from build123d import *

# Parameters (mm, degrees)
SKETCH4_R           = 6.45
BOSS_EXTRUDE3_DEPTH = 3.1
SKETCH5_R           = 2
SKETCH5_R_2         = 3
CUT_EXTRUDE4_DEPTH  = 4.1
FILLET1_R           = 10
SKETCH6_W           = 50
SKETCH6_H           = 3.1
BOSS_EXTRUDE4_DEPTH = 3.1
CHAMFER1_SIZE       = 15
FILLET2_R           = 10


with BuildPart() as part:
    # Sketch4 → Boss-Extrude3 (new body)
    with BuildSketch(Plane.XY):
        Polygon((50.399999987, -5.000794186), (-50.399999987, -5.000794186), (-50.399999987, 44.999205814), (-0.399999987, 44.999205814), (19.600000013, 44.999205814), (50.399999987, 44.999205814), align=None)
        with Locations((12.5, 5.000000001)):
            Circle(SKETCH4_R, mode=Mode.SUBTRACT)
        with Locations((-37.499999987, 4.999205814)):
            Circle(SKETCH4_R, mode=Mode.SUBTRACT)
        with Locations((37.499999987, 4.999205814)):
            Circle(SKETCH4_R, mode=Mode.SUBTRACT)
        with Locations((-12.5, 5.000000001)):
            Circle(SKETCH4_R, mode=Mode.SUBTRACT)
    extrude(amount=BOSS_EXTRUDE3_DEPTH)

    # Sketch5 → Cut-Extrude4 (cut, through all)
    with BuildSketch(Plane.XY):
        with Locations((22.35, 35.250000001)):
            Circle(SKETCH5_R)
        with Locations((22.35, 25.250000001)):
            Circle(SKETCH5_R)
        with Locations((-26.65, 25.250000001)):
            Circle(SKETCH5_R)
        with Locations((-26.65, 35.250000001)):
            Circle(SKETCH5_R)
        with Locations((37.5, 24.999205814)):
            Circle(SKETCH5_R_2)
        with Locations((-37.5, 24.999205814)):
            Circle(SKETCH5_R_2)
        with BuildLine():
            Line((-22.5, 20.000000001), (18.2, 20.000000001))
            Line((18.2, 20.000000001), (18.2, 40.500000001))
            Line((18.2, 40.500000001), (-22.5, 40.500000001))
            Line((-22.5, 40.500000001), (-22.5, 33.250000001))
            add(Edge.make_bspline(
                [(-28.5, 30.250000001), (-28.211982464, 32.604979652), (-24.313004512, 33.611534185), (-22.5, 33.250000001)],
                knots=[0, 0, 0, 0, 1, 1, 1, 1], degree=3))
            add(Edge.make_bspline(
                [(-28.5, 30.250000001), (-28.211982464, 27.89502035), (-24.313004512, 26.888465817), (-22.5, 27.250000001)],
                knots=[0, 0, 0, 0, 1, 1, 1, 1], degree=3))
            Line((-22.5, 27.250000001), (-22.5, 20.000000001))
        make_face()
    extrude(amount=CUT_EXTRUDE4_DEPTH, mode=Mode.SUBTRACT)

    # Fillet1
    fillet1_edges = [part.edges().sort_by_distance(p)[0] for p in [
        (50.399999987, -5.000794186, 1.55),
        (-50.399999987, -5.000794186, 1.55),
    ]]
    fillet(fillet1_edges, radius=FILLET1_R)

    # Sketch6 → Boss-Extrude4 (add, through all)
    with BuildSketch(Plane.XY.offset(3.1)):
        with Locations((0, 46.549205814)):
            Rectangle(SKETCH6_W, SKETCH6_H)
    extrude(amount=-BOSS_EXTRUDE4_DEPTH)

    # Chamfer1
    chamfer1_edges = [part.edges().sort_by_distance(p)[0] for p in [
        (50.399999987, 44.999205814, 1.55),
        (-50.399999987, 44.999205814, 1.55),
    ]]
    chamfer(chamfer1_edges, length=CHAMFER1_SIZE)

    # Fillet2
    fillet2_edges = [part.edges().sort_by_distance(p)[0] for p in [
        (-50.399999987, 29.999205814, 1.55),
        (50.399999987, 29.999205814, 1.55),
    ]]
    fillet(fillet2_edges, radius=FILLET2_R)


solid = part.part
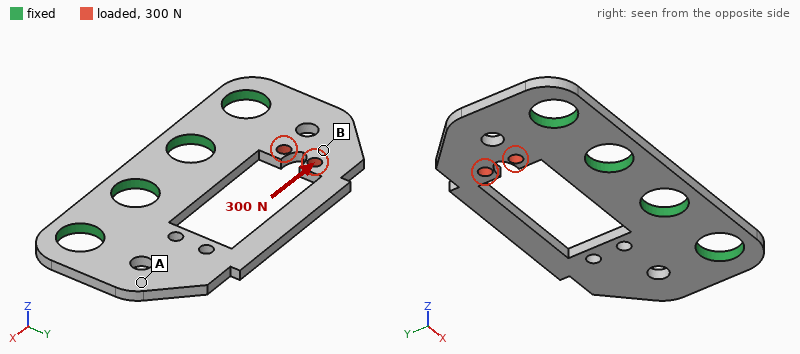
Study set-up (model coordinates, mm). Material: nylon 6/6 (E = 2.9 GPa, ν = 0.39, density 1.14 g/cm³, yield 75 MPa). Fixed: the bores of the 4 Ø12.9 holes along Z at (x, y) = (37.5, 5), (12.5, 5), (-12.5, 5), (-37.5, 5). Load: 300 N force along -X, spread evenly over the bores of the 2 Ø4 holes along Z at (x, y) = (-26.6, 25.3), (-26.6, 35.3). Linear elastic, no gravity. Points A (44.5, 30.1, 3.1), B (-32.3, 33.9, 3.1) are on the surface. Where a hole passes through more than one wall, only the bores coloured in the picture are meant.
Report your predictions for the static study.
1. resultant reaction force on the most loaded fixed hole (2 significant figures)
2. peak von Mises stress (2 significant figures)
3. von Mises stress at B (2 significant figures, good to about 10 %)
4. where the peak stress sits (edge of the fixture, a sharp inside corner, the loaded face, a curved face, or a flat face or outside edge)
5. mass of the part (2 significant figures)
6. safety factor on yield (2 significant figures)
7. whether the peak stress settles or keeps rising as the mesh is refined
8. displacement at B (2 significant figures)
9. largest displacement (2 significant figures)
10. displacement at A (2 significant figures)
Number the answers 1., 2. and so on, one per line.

1. 170 N
2. 29 MPa
3. 5.3 MPa
4. the loaded face
5. 12 g
6. 2.5
7. settles
8. 0.11 mm
9. 0.14 mm
10. 0.032 mm
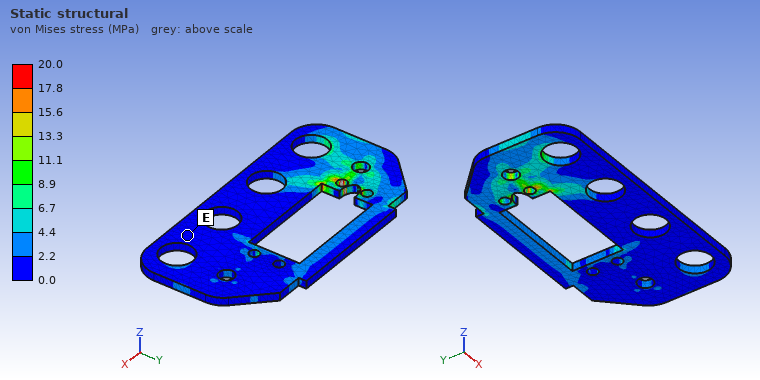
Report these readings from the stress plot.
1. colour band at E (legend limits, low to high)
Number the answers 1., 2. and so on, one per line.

1. 0.0 to 2.2 MPa
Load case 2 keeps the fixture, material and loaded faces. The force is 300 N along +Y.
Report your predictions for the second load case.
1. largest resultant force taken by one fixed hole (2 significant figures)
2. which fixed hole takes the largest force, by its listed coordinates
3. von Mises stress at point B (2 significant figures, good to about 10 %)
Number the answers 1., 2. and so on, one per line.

1. 230 N
2. (-37.5, 5)
3. 4.9 MPa
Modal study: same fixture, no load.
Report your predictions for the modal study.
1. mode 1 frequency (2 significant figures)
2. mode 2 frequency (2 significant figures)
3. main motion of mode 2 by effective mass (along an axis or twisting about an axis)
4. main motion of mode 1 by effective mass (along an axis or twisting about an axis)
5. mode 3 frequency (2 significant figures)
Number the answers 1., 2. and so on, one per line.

1. 520 Hz
2. 870 Hz
3. twisting about Y
4. along Z
5. 1400 Hz
